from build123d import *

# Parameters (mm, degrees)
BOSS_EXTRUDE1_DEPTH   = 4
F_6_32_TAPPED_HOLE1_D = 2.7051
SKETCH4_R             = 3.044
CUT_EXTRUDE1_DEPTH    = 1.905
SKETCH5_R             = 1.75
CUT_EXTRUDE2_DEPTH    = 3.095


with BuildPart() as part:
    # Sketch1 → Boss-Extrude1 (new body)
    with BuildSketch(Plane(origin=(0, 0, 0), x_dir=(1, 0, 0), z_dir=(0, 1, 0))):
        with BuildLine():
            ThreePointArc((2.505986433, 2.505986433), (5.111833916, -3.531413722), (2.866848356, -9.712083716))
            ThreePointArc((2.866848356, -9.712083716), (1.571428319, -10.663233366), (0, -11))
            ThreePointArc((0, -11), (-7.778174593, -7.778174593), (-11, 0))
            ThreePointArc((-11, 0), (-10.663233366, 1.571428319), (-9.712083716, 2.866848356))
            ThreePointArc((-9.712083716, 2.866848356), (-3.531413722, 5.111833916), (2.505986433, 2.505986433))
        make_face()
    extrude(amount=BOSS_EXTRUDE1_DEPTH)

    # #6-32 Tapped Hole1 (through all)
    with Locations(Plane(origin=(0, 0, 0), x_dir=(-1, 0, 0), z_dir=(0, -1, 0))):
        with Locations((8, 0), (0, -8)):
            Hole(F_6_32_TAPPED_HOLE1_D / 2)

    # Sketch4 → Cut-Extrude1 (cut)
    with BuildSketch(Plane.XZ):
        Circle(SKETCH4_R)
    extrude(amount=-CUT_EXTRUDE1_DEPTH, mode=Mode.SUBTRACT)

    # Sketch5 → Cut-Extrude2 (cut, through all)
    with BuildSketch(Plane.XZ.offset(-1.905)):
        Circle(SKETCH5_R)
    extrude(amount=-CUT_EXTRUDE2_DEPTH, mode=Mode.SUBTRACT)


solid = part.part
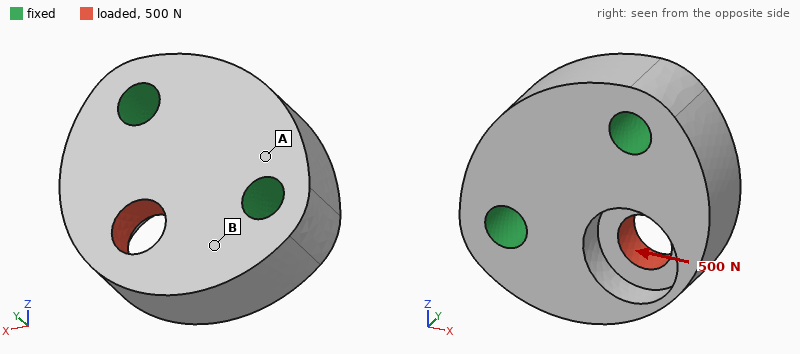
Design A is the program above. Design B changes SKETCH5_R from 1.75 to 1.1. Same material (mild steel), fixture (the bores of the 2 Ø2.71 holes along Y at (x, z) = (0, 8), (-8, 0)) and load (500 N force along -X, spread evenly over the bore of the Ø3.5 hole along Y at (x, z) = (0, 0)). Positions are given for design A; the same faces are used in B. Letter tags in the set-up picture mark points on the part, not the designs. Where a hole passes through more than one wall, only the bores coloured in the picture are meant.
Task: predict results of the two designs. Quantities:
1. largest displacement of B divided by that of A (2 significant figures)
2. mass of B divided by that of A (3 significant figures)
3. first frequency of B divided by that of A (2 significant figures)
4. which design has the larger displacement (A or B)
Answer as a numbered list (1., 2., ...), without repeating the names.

1. 0.85
2. 1.02
3. 0.98
4. A
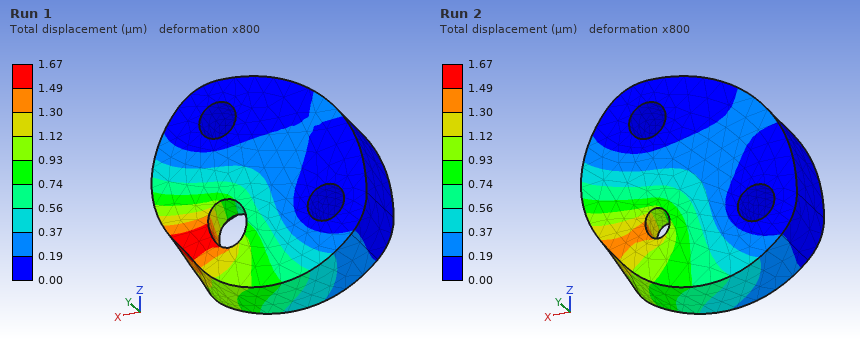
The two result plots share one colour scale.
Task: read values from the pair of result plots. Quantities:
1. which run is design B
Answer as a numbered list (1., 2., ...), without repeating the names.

1. Run 2
